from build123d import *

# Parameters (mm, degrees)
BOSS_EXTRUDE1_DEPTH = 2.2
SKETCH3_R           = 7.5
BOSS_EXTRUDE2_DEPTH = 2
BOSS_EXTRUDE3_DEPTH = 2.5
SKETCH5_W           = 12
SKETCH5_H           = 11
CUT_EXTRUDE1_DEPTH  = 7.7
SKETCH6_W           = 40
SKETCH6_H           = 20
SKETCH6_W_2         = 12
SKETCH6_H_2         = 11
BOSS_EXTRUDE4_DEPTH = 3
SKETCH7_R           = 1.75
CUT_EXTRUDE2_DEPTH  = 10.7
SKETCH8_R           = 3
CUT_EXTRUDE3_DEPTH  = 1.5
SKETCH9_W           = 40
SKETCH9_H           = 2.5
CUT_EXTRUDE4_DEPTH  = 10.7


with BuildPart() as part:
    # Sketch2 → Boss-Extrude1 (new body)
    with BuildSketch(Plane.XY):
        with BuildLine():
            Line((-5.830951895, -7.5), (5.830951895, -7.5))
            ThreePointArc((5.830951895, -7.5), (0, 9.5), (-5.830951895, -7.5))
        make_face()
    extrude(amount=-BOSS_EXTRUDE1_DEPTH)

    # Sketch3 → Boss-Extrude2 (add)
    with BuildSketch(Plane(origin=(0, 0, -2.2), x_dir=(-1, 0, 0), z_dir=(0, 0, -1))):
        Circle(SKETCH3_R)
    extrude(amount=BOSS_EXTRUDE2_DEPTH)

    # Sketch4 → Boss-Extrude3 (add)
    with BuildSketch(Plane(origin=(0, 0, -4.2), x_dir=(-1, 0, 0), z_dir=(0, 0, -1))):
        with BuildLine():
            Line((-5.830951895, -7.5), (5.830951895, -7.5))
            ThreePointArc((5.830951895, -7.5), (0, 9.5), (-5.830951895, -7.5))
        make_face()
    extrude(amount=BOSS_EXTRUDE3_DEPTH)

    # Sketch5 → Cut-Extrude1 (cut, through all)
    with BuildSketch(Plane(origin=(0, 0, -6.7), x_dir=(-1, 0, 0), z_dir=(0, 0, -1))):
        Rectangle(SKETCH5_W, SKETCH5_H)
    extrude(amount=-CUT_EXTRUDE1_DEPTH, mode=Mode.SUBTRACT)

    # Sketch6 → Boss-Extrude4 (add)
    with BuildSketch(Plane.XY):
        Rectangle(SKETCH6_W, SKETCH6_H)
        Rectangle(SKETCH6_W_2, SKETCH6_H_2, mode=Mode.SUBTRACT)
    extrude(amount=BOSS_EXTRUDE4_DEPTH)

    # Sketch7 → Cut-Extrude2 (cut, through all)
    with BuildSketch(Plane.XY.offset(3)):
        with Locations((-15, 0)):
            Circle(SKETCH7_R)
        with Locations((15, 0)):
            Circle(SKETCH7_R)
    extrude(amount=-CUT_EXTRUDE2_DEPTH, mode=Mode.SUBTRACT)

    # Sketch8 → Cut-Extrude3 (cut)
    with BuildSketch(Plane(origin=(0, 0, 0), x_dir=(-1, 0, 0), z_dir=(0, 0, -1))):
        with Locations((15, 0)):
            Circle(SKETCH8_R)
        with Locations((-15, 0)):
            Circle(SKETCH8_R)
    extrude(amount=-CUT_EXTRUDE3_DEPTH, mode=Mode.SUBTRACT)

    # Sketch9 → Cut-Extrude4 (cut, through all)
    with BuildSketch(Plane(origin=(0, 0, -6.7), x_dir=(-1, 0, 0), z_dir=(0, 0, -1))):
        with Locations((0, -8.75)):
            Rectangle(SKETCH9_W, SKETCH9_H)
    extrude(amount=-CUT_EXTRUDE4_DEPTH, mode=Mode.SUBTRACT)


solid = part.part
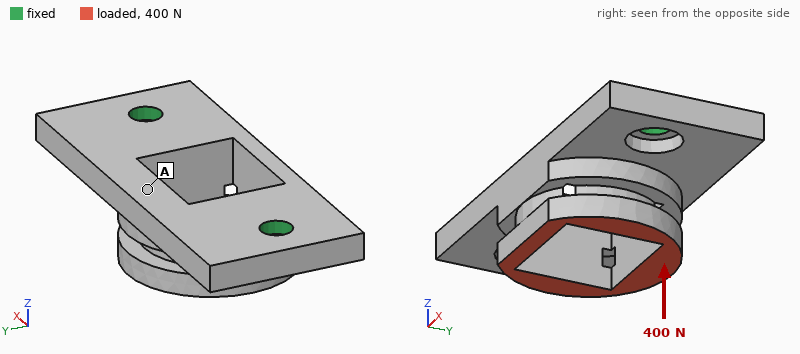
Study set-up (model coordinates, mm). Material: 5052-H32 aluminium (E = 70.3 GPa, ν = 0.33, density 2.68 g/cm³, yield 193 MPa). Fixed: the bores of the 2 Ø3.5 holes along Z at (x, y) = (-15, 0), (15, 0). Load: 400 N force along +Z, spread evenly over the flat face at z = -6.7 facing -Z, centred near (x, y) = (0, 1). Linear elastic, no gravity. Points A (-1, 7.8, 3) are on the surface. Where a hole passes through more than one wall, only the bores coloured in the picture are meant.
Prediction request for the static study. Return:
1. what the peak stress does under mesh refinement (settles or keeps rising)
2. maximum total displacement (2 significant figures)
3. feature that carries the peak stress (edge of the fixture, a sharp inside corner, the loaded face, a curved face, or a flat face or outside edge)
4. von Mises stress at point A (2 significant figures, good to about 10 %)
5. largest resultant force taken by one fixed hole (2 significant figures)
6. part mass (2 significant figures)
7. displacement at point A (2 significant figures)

keeps rising
25 µm
edge of the fixture
15 MPa
290 N
6.2 g
20 µm
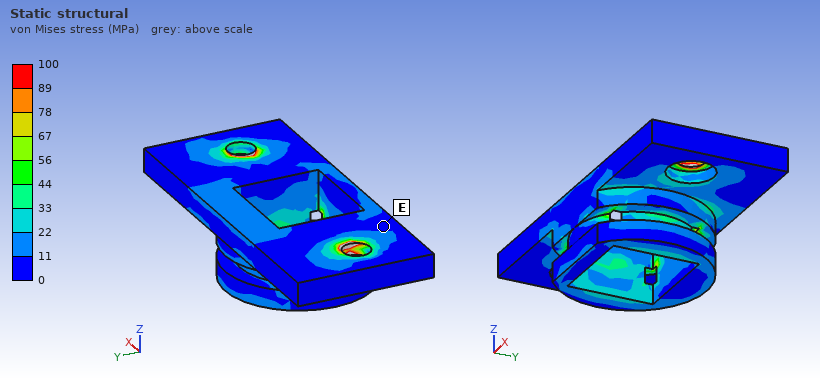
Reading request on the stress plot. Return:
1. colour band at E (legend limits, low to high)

0 to 11 MPa
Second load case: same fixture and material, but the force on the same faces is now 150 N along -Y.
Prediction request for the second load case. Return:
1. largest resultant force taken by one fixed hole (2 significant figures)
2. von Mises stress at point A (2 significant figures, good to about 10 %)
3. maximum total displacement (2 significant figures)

78 N
9.3 MPa
33 µm
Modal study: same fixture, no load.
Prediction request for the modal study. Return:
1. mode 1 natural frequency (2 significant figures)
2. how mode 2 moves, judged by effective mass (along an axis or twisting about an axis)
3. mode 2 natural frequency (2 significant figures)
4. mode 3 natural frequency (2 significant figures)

8200 Hz
along Z
14 kHz
19 kHz
